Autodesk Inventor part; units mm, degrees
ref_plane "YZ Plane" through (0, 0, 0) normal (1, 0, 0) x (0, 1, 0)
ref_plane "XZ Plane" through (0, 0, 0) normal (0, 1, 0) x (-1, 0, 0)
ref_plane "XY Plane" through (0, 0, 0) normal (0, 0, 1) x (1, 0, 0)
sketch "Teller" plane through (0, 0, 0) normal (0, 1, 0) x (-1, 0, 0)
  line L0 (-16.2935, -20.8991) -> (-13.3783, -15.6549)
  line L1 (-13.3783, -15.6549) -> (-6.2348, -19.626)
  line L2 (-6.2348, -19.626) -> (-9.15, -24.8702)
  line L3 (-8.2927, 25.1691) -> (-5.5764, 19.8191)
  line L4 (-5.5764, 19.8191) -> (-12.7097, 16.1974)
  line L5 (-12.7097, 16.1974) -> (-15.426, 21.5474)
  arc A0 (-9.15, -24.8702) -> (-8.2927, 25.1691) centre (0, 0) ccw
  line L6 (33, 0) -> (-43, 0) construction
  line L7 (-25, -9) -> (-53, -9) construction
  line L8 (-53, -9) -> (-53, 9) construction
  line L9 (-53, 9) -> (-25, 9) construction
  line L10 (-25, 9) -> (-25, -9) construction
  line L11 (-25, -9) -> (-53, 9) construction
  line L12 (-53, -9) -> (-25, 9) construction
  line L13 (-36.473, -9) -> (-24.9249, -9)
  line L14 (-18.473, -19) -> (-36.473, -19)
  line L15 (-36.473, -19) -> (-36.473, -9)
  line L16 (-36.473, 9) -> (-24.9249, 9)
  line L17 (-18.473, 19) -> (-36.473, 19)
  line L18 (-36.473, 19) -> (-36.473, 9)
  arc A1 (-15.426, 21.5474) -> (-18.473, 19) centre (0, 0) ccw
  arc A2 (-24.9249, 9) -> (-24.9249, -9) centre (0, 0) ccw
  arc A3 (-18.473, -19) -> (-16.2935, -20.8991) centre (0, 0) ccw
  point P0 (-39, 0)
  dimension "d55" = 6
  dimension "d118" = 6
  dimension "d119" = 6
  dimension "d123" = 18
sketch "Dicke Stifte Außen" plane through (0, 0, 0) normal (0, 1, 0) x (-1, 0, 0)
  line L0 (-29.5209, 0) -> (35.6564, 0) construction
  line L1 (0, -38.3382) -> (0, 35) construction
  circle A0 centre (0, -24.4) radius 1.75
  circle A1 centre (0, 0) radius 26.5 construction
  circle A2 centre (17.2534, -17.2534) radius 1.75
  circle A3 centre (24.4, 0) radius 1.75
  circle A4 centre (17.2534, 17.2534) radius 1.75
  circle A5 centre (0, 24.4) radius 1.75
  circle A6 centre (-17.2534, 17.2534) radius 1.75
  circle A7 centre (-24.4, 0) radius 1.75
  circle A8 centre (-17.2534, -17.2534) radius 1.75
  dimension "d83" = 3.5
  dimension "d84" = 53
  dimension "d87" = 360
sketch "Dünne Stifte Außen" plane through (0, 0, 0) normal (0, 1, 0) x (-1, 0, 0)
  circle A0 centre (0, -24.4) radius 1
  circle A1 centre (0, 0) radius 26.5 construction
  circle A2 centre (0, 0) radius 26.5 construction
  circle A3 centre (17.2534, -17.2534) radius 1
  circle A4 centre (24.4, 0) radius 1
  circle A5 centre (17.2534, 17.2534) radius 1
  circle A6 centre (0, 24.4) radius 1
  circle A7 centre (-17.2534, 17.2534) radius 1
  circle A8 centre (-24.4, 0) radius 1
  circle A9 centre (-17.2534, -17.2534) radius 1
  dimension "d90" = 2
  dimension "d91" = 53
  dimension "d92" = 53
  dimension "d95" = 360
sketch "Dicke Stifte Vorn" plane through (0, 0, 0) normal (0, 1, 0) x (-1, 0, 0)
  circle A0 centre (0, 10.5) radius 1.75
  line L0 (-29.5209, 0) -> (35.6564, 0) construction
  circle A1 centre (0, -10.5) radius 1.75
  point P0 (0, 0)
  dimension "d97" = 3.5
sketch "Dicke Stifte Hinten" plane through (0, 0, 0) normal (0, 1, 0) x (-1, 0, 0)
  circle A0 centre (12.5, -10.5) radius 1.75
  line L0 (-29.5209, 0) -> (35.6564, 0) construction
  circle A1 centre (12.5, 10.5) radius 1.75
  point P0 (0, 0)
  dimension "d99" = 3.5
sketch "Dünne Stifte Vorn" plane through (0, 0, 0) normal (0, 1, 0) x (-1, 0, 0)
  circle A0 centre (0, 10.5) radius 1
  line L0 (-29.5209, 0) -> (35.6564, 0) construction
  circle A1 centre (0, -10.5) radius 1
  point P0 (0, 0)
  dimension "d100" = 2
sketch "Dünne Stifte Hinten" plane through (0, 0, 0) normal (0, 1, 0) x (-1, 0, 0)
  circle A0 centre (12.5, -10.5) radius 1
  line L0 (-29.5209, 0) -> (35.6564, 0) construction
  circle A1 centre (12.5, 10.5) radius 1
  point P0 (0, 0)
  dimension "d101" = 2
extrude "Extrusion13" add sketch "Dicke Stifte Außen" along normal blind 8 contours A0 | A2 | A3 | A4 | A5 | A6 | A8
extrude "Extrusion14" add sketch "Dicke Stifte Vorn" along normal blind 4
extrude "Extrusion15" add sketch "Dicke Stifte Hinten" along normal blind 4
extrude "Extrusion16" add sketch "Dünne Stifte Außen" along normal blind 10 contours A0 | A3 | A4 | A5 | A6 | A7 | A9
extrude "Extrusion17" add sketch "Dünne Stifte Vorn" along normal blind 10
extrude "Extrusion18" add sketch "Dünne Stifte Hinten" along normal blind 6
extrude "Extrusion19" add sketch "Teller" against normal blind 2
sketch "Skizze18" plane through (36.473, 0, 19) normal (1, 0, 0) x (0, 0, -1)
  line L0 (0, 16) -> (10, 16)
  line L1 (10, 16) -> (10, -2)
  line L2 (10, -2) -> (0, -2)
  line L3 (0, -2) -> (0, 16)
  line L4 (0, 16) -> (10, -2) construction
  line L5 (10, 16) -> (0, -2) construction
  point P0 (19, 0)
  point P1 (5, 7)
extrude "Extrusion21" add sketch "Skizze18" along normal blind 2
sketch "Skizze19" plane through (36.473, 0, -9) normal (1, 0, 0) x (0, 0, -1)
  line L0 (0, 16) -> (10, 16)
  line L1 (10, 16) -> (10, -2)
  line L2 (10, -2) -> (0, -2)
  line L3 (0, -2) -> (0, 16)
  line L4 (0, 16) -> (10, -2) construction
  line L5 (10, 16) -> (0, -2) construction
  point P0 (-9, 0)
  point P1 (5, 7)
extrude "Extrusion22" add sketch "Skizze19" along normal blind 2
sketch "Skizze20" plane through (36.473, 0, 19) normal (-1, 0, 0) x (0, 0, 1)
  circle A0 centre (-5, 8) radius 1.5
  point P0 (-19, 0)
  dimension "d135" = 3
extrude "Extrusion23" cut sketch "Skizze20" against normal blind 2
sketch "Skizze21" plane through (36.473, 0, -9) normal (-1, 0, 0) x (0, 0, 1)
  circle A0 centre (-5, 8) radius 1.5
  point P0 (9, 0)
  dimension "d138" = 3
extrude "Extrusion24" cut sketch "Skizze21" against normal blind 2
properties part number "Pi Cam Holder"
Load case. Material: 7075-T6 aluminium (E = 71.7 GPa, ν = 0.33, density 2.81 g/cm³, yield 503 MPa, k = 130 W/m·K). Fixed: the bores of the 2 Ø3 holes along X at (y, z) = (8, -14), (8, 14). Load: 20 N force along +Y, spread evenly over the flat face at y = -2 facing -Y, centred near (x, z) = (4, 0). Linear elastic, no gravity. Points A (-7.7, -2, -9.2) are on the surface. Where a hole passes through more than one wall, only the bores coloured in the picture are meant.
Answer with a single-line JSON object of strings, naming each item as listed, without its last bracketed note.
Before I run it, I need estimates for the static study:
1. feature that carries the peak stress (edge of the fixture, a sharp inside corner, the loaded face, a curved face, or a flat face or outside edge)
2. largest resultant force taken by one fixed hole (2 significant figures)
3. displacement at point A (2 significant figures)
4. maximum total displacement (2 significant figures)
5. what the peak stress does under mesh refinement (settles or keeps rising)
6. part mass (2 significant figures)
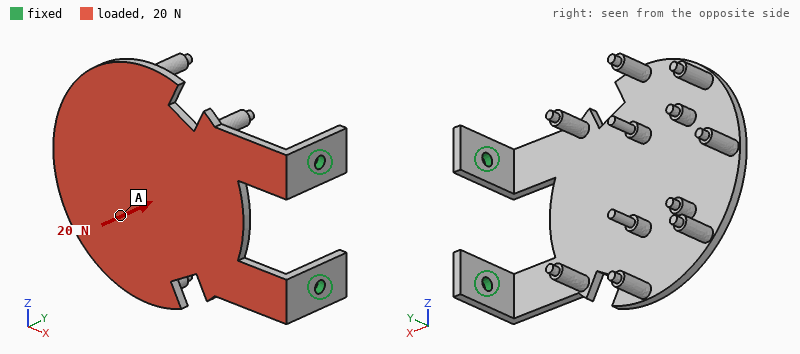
{"feature that carries the peak stress": "edge of the fixture", "largest resultant force taken by one fixed hole": "10 N", "displacement at point A": "0.62 mm", "maximum total displacement": "0.93 mm", "what the peak stress does under mesh refinement": "keeps rising", "part mass": "18 g"}
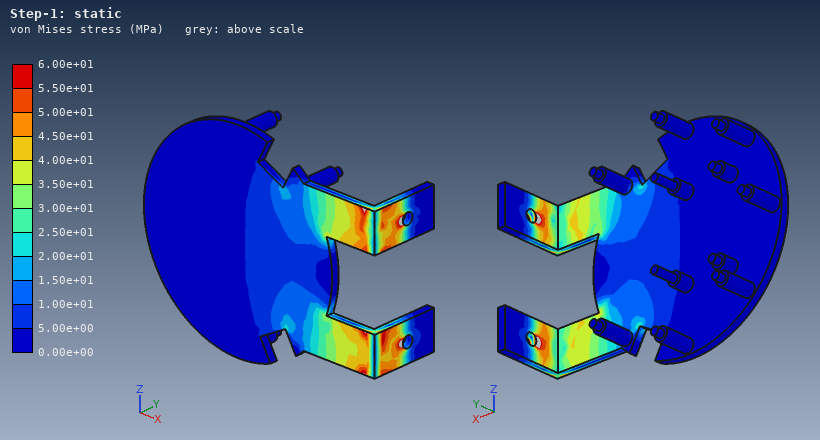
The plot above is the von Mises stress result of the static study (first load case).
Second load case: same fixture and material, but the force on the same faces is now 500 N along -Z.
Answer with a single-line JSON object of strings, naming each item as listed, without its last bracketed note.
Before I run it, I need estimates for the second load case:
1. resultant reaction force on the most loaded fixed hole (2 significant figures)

{"resultant reaction force on the most loaded fixed hole": "580 N"}
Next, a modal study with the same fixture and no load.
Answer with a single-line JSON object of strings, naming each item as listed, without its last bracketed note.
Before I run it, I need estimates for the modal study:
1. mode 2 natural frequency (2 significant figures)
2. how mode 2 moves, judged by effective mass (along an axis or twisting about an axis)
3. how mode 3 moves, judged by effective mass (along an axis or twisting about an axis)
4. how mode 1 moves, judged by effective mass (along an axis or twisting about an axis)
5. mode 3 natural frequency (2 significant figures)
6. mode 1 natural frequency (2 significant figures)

{"mode 2 natural frequency": "830 Hz", "how mode 2 moves, judged by effective mass": "along Z", "how mode 3 moves, judged by effective mass": "along Z", "how mode 1 moves, judged by effective mass": "along Y", "mode 3 natural frequency": "1300 Hz", "mode 1 natural frequency": "230 Hz"}
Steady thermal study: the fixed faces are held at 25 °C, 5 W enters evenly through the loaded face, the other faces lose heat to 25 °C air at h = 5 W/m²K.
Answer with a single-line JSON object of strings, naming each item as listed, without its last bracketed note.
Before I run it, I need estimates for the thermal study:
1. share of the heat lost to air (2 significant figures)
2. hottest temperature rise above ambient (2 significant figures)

{"share of the heat lost to air": "9.6 %", "hottest temperature rise above ambient": "29 K"}
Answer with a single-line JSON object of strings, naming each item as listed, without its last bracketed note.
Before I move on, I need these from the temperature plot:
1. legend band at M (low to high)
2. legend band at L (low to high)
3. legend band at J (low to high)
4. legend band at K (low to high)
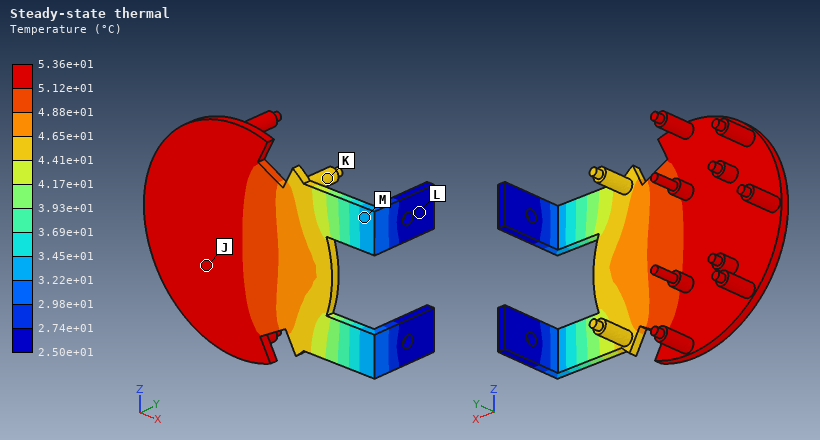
{"legend band at M": "3.22e+01 to 3.45e+01 °C", "legend band at L": "2.50e+01 to 2.74e+01 °C", "legend band at J": "5.12e+01 to 5.36e+01 °C", "legend band at K": "4.41e+01 to 4.65e+01 °C"}
